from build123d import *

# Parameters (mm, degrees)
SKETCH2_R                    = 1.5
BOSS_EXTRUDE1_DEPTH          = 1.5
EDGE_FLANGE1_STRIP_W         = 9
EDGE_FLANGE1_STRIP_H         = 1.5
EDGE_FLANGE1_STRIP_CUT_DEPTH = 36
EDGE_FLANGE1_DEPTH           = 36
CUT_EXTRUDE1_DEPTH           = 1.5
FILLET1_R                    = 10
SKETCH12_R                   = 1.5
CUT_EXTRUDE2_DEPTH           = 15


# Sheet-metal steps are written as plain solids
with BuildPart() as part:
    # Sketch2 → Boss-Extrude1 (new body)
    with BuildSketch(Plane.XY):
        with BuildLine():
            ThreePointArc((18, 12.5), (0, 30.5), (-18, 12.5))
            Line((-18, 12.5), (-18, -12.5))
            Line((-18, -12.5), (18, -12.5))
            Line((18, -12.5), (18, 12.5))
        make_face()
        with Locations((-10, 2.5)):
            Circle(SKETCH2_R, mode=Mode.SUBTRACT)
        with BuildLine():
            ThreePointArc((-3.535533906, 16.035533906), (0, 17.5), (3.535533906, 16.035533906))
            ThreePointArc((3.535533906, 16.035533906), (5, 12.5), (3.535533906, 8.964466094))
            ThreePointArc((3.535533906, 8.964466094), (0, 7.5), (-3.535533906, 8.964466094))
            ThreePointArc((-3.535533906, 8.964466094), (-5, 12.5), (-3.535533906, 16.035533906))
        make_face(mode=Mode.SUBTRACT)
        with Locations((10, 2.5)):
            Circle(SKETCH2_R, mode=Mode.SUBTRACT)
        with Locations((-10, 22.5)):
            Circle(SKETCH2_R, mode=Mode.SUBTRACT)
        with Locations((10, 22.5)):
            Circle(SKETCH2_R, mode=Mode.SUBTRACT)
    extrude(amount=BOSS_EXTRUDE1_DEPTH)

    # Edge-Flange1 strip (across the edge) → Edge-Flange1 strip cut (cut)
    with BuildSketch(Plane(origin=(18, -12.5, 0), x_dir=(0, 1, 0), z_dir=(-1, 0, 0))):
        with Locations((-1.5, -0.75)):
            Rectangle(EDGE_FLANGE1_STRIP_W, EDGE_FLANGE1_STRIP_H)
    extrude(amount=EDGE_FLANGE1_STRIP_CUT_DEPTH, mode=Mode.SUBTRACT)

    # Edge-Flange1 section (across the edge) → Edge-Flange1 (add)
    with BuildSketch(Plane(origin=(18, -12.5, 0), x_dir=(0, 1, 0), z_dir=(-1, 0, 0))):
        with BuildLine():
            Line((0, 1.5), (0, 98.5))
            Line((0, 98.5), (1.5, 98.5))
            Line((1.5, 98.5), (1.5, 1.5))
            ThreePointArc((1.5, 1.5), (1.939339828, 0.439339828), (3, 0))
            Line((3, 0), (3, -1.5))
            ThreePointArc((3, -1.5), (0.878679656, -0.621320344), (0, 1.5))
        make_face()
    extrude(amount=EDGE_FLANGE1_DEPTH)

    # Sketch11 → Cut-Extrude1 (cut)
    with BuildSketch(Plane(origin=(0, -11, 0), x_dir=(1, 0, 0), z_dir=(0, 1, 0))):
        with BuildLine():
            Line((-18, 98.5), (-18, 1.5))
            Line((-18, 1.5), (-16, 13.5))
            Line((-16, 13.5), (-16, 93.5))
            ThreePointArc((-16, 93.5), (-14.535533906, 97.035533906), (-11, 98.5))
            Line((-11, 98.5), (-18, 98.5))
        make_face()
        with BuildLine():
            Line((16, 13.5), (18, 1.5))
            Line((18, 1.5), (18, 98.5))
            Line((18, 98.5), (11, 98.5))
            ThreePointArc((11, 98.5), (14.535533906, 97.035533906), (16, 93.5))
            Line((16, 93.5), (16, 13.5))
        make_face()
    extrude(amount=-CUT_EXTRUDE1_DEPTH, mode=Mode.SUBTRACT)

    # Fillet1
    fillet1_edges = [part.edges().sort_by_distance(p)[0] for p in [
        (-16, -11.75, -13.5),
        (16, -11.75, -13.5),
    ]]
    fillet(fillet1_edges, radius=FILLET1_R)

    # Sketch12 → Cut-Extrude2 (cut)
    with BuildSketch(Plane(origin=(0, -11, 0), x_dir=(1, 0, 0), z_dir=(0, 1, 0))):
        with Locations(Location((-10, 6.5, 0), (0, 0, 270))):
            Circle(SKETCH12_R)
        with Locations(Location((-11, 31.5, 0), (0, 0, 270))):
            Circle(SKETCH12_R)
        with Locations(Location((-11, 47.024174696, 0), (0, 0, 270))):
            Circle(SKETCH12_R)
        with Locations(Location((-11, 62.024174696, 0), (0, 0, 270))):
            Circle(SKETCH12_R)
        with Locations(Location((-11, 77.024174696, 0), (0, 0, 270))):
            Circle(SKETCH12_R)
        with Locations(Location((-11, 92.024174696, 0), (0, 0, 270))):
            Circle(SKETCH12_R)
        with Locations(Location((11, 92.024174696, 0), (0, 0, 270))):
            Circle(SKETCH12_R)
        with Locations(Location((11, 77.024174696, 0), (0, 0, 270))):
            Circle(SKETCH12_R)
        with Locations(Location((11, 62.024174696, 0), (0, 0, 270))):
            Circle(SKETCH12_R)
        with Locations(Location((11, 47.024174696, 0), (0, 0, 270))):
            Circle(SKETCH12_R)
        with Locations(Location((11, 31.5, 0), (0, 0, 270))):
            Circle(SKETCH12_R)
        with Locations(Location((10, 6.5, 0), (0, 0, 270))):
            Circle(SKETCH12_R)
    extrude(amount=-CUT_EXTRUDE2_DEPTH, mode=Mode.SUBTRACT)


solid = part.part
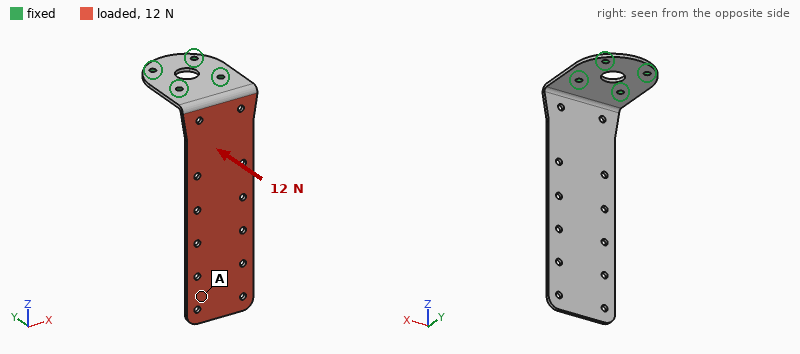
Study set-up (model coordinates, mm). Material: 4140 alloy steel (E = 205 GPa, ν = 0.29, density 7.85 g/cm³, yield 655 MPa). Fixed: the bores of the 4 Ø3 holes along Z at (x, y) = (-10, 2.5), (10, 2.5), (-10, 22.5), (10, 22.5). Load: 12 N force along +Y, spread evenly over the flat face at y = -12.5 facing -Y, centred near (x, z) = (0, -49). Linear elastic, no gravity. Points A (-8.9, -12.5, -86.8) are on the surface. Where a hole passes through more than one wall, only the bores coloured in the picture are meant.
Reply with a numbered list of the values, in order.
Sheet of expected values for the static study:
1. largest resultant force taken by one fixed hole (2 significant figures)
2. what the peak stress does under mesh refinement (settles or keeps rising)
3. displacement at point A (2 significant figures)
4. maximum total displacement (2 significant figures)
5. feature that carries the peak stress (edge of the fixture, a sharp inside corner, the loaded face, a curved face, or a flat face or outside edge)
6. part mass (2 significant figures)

1. 7.3 N
2. keeps rising
3. 0.98 mm
4. 1.2 mm
5. edge of the fixture
6. 51 g
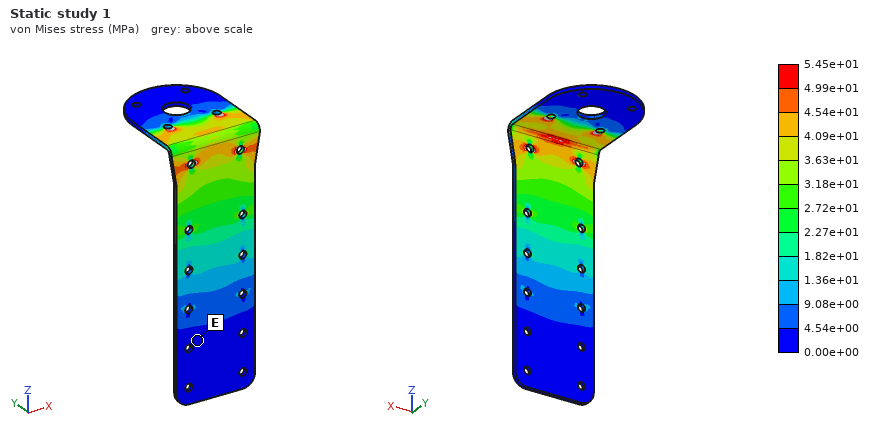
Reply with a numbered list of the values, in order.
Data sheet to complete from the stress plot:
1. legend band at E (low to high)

1. 0.00e+00 to 4.54e+00 MPa
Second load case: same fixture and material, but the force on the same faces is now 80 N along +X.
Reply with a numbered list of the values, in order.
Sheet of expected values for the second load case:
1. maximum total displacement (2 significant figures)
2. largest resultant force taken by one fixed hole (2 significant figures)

1. 0.62 mm
2. 190 N
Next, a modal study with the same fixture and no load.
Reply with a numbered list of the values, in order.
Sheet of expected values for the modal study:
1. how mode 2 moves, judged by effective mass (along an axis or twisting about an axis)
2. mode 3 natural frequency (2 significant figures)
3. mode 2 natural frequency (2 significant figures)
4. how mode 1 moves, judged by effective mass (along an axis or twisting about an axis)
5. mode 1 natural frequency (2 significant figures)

1. along X
2. 670 Hz
3. 360 Hz
4. along Y
5. 110 Hz
